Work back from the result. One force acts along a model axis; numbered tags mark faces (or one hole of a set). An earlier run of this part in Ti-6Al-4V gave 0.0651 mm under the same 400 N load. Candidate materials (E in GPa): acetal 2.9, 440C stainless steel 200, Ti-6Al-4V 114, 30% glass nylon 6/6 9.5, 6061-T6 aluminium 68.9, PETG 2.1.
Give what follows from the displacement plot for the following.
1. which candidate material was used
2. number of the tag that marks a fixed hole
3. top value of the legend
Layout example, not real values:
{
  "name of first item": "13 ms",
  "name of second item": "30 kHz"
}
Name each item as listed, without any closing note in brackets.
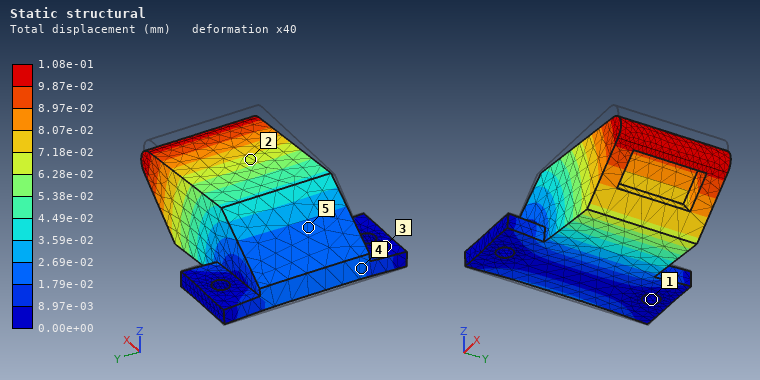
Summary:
{
  "which candidate material was used": "6061-T6 aluminium",
  "number of the tag that marks a fixed hole": "1",
  "top value of the legend": "1.08e-01 mm"
}
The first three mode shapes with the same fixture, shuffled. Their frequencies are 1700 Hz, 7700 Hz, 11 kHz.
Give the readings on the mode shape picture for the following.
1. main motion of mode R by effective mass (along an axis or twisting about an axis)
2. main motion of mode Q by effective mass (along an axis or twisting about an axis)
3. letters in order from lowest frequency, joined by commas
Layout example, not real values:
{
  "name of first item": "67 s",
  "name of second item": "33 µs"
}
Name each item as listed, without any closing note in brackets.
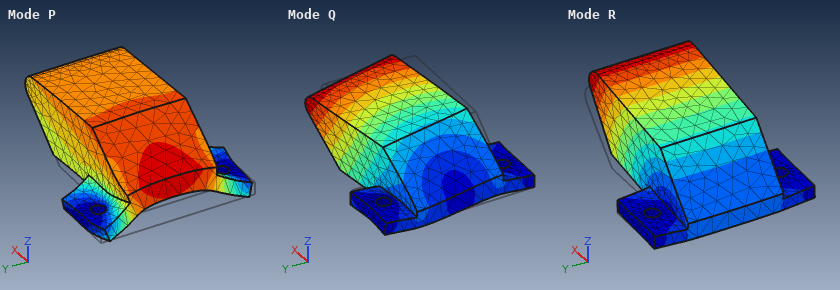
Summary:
{
  "main motion of mode R by effective mass": "along Z",
  "main motion of mode Q by effective mass": "along Y",
  "letters in order from lowest frequency, joined by commas": "R, Q, P"
}
